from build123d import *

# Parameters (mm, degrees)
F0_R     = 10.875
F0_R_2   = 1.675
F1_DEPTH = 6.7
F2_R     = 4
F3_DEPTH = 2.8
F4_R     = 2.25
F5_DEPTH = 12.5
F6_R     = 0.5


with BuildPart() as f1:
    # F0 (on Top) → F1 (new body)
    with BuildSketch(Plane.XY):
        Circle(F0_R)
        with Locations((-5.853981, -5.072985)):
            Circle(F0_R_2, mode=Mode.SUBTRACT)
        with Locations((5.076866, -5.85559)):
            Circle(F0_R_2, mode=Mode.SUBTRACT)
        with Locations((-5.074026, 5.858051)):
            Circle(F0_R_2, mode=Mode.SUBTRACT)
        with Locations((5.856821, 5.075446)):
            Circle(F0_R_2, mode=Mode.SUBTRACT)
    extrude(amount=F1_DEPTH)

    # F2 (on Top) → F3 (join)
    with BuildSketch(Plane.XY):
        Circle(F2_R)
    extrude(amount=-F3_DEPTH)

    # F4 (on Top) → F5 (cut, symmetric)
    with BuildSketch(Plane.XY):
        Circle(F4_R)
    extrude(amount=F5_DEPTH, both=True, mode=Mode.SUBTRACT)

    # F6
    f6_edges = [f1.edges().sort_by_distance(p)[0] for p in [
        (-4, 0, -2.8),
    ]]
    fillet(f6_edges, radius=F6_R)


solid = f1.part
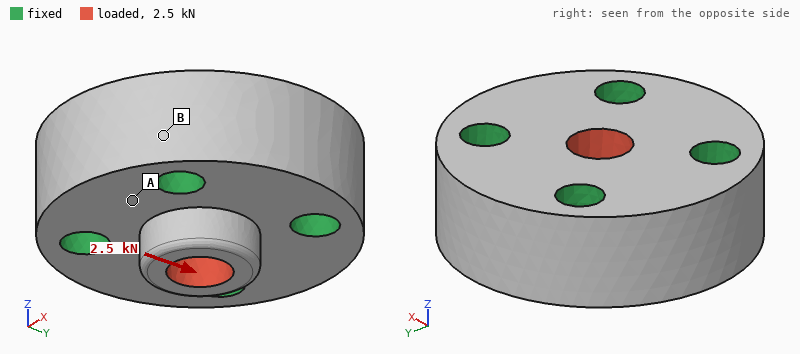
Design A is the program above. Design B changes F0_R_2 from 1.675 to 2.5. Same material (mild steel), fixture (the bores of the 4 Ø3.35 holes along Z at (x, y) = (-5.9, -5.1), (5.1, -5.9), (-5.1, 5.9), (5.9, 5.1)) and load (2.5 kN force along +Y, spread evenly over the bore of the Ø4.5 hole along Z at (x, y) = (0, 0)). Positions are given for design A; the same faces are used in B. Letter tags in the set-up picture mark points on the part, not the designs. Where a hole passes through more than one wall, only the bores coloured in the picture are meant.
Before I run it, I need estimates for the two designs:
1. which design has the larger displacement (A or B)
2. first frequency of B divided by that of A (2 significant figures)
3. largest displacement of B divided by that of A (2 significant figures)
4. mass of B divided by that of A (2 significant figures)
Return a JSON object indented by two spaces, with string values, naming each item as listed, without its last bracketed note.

{
  "which design has the larger displacement": "A",
  "first frequency of B divided by that of A": "1.3",
  "largest displacement of B divided by that of A": "0.92",
  "mass of B divided by that of A": "0.87"
}
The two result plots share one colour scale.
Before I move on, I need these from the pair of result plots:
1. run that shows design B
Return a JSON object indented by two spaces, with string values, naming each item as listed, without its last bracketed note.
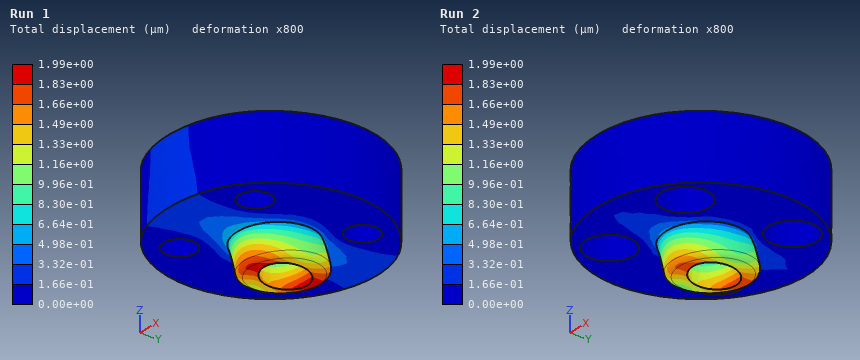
{
  "run that shows design B": "Run 2"
}
